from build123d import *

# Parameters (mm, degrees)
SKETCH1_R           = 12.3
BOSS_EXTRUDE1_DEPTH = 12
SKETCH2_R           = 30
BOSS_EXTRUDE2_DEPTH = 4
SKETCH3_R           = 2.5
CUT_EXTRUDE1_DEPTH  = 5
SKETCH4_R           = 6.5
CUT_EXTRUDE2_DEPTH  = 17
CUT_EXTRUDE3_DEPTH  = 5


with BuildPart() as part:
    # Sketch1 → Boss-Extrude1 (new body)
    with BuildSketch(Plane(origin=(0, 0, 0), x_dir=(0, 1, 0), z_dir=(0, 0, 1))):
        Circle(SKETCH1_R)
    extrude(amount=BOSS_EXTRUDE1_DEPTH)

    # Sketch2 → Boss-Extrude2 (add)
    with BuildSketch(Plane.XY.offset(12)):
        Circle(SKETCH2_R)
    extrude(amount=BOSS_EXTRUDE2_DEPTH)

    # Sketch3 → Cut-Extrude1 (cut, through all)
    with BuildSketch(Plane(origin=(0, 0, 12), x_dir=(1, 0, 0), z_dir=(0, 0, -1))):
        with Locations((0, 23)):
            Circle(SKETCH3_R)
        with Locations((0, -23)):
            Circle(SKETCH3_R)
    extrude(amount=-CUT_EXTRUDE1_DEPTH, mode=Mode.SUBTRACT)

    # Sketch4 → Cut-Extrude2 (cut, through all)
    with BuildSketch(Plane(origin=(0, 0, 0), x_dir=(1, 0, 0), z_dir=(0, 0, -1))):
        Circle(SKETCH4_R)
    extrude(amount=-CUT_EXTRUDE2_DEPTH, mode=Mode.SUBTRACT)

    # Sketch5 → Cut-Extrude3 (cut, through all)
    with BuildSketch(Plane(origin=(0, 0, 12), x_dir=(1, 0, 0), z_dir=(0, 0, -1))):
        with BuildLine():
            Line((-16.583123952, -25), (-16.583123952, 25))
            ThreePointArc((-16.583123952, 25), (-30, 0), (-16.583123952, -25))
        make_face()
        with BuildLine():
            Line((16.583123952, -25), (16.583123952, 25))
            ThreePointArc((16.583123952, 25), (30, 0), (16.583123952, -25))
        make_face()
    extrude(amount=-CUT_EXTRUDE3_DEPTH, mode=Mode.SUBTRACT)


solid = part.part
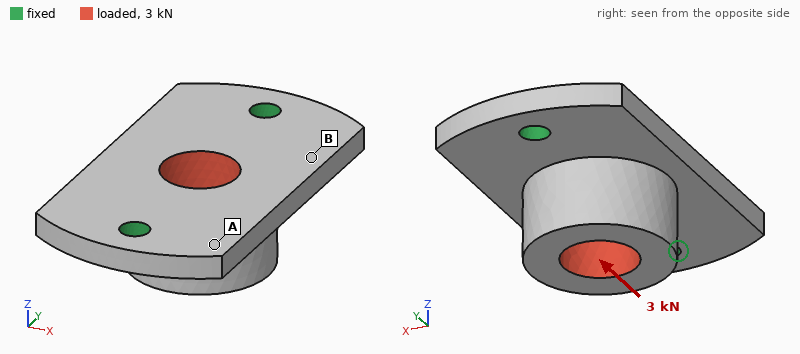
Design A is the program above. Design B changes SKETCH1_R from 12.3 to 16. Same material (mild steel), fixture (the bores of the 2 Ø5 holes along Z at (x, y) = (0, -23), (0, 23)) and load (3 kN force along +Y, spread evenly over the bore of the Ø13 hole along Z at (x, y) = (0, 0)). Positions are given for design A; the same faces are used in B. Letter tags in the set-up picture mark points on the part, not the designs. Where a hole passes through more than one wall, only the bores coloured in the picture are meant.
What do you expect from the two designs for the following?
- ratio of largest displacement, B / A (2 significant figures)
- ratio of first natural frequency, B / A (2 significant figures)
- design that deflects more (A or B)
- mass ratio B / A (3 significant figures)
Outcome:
0.46
0.88
A
1.36
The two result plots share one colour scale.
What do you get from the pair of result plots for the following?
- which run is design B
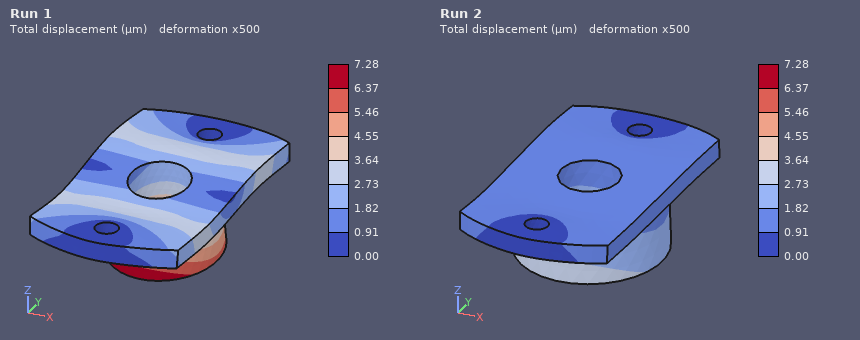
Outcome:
Run 2
